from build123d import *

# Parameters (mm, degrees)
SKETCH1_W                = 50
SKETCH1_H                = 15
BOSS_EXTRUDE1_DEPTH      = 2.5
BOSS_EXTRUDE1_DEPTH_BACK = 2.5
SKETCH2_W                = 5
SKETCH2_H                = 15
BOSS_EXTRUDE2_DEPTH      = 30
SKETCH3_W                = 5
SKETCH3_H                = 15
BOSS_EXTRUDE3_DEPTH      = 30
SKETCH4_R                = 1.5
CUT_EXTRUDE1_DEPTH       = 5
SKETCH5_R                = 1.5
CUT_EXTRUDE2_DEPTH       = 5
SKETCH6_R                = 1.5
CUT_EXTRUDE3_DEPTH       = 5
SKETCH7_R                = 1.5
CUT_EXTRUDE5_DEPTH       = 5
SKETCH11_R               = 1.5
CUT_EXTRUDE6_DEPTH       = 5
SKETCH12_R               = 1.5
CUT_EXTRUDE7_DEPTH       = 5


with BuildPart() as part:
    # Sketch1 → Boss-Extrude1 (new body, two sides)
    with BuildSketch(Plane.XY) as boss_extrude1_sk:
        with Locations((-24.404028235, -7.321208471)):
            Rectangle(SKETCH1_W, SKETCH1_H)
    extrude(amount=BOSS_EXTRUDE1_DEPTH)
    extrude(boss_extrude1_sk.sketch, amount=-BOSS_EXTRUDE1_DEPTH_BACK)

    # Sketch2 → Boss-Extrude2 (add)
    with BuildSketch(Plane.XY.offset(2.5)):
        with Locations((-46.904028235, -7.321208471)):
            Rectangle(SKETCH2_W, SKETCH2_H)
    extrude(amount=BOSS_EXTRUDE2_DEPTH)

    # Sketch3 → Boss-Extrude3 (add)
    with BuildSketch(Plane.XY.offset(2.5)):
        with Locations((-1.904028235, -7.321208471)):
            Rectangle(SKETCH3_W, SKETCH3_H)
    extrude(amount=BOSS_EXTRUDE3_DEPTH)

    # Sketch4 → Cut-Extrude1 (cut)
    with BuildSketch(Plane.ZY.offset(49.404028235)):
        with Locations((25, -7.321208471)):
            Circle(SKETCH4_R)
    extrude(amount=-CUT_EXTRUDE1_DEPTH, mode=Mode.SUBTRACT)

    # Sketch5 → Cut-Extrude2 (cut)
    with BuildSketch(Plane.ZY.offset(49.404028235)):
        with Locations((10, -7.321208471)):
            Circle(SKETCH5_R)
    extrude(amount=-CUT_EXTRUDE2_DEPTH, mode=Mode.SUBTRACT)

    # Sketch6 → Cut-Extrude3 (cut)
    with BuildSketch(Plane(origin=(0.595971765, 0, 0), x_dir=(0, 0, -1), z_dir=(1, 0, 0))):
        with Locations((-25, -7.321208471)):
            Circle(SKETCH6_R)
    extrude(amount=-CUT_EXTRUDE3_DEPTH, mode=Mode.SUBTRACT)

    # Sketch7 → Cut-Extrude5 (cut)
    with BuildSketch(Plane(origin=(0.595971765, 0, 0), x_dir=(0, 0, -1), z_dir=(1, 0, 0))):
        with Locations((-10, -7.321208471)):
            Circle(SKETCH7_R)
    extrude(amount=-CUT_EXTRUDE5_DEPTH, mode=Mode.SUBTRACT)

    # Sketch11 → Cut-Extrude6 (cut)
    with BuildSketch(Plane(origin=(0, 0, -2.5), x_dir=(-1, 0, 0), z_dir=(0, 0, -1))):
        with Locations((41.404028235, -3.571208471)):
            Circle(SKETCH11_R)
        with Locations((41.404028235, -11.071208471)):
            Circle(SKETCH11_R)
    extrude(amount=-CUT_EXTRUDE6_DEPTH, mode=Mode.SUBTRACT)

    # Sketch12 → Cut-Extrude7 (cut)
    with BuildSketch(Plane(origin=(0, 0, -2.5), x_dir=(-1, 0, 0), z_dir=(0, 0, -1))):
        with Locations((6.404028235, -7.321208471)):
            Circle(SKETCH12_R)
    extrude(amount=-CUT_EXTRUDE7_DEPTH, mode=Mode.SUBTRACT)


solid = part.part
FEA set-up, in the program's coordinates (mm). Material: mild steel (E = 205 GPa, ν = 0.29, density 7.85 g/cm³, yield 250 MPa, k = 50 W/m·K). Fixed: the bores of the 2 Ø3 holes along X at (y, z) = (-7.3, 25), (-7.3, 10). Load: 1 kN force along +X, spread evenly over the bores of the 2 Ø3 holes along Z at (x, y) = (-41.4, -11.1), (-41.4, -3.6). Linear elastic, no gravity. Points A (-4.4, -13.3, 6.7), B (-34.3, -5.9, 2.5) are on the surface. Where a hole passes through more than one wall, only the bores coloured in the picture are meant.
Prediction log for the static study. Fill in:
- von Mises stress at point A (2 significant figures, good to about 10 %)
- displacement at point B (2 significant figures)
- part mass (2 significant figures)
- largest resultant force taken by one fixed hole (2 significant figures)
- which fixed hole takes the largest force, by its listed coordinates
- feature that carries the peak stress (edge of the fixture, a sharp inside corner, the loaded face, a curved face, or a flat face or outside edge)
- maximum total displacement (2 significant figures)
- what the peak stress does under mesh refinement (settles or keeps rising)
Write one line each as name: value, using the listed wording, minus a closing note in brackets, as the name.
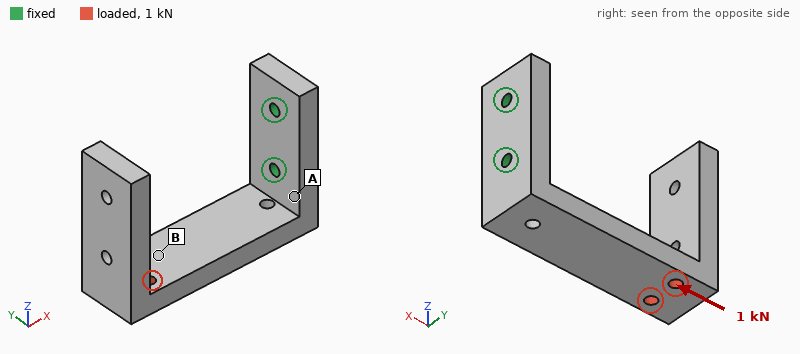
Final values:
von Mises stress at point A: 79 MPa
displacement at point B: 57 µm
part mass: 63 g
largest resultant force taken by one fixed hole: 1.2 kN
which fixed hole takes the largest force, by its listed coordinates: (-7.3, 10)
feature that carries the peak stress: edge of the fixture
maximum total displacement: 91 µm
what the peak stress does under mesh refinement: keeps rising
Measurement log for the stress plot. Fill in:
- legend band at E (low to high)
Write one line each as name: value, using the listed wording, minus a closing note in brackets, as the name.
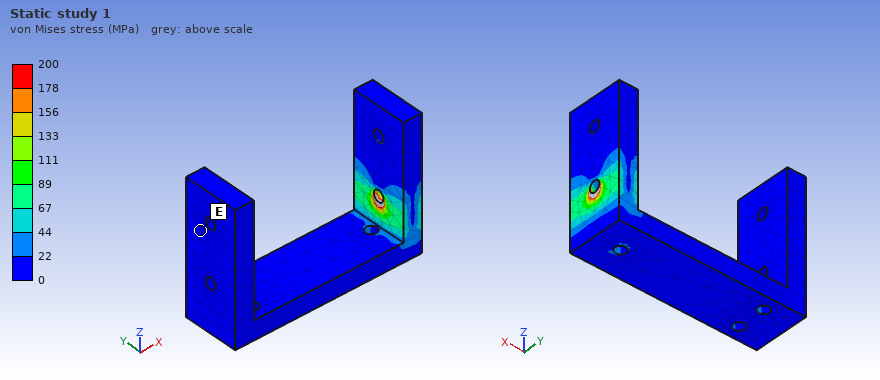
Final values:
legend band at E: 0 to 22 MPa
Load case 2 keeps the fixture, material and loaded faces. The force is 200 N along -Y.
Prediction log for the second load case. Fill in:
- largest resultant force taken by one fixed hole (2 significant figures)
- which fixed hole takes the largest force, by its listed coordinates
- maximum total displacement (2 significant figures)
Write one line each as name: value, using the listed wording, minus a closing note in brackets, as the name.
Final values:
largest resultant force taken by one fixed hole: 290 N
which fixed hole takes the largest force, by its listed coordinates: (-7.3, 10)
maximum total displacement: 0.11 mm
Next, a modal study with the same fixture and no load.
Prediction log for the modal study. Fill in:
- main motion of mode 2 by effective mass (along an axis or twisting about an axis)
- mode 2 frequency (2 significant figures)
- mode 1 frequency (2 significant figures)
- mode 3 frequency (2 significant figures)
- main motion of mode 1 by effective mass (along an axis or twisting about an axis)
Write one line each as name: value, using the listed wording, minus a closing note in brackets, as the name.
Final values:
main motion of mode 2 by effective mass: along Y
mode 2 frequency: 1100 Hz
mode 1 frequency: 730 Hz
mode 3 frequency: 2300 Hz
main motion of mode 1 by effective mass: along Z
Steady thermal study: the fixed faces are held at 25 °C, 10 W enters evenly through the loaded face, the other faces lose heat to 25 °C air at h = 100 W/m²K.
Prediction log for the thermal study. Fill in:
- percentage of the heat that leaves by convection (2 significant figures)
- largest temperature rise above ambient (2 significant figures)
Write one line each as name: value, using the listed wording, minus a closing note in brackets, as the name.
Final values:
percentage of the heat that leaves by convection: 79 %
largest temperature rise above ambient: 41 K
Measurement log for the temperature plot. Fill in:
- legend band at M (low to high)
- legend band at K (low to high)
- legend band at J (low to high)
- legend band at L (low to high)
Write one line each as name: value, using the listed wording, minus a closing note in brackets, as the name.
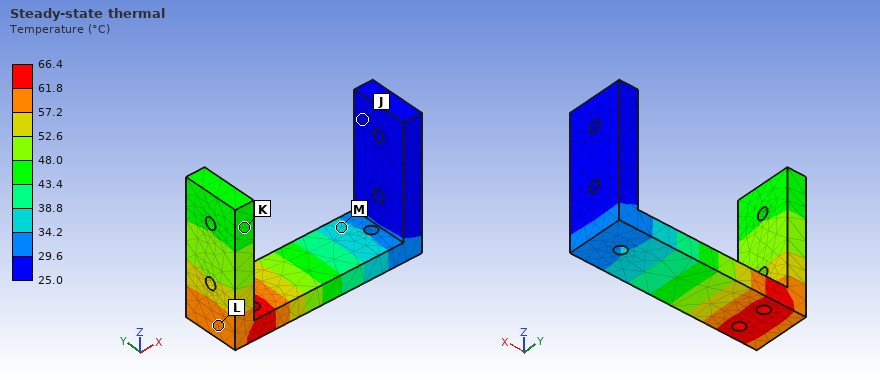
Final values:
legend band at M: 34.2 to 38.8 °C
legend band at K: 43.4 to 48.0 °C
legend band at J: 25.0 to 29.6 °C
legend band at L: 57.2 to 61.8 °C
